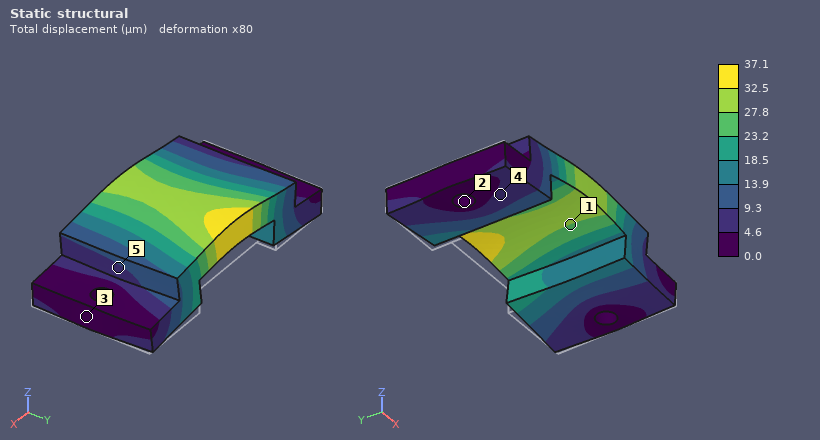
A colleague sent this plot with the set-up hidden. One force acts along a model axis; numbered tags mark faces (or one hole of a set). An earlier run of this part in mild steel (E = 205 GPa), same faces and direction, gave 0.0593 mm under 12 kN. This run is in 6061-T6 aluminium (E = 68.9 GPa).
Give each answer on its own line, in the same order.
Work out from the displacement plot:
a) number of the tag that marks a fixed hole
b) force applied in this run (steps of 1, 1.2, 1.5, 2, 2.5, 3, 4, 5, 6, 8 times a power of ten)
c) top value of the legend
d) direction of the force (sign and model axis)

2
2.5 kN
37.1 µm
+Z
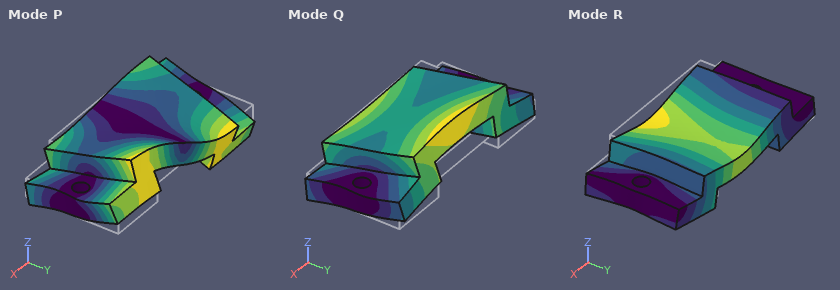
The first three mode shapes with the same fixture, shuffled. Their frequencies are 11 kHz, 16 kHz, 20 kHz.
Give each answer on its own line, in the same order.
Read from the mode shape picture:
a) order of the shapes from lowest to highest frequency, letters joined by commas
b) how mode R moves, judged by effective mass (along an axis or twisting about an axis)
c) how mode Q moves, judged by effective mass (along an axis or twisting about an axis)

Q, R, P
along Z
along Y
